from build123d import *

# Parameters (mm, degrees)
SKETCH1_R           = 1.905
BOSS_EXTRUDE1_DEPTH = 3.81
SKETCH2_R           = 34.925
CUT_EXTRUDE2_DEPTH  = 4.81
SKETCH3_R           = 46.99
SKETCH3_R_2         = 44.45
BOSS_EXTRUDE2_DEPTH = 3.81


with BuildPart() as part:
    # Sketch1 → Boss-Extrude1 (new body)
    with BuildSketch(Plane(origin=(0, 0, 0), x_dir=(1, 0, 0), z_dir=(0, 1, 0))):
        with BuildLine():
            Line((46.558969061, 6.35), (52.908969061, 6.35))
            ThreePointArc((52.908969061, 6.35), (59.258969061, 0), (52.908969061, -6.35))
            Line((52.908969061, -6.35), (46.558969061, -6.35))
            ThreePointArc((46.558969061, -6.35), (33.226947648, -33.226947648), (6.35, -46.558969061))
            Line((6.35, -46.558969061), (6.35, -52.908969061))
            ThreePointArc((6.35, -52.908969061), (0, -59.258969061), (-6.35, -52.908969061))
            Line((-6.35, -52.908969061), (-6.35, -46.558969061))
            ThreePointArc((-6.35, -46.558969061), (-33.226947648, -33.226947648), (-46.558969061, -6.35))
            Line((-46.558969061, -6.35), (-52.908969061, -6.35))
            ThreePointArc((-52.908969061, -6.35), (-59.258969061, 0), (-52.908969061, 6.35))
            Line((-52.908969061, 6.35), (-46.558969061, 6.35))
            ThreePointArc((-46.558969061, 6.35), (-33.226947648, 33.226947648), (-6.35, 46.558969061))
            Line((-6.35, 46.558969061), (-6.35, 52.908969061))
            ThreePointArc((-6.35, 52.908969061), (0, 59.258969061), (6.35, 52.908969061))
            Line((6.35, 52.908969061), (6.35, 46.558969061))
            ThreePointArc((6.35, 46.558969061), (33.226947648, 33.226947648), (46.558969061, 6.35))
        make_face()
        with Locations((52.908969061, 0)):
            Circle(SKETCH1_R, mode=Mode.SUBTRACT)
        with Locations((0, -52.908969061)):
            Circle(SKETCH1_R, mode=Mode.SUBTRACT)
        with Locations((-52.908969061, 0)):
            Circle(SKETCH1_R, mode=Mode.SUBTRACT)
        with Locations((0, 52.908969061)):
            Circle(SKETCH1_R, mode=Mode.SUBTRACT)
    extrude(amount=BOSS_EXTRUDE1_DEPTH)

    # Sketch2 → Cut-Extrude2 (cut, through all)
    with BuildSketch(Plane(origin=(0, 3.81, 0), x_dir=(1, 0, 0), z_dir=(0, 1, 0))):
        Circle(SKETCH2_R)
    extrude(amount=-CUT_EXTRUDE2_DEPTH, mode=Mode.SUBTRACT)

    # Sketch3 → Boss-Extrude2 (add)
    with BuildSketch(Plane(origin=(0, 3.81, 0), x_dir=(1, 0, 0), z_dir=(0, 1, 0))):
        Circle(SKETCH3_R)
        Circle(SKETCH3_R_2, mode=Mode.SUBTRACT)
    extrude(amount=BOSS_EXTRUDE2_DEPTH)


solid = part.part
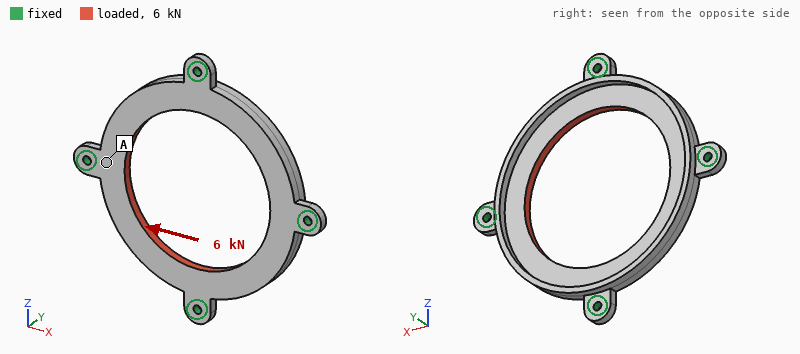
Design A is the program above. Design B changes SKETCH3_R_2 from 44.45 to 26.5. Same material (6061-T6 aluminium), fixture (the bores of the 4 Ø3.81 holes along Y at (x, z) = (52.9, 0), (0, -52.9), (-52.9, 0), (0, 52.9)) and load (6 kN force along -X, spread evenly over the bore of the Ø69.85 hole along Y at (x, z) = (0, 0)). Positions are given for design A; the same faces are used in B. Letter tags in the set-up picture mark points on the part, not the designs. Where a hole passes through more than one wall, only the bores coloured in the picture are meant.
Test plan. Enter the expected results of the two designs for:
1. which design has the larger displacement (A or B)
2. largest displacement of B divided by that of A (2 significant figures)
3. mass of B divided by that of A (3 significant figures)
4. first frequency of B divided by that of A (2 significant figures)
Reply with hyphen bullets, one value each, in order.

- A
- 0.54
- 1.92
- 1.2
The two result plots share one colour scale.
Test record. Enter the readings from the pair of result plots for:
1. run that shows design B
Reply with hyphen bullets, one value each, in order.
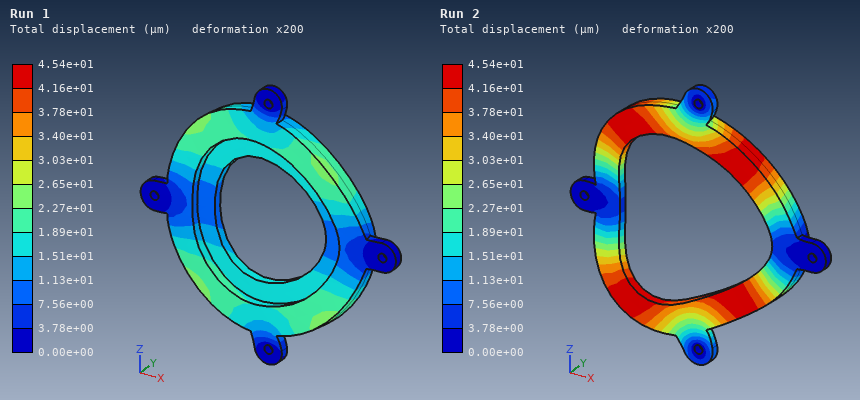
- Run 1
